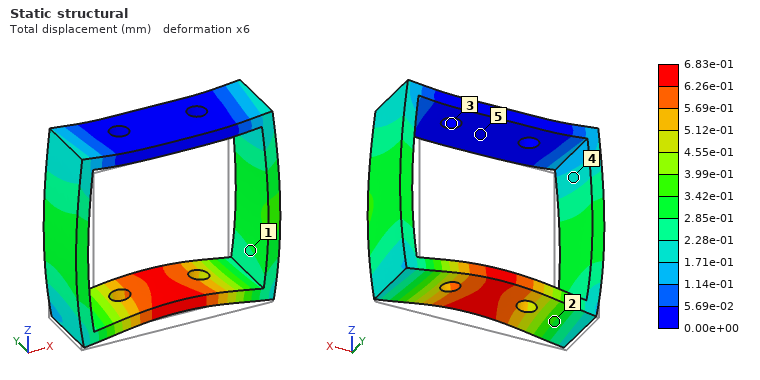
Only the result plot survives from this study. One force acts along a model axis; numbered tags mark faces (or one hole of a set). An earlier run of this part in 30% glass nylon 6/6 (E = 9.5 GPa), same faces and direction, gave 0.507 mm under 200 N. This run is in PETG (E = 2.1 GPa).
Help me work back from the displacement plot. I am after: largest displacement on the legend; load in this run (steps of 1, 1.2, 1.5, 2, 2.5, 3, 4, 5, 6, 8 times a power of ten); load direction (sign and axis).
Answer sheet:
6.83e-01 mm
60 N
+Z
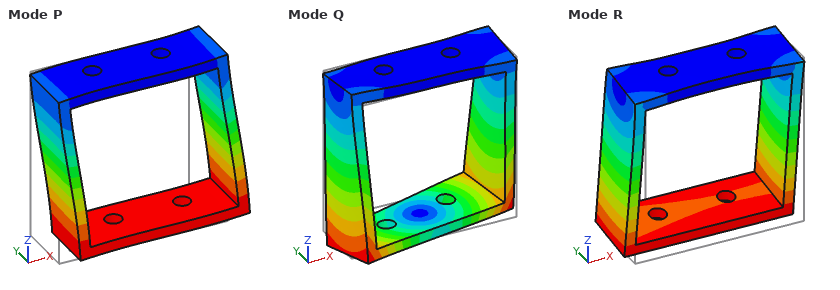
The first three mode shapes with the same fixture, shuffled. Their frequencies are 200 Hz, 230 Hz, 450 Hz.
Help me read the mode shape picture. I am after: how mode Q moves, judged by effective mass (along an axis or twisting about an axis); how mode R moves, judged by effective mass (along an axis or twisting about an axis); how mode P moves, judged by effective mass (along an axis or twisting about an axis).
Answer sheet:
twisting about Z
along Y
along X
